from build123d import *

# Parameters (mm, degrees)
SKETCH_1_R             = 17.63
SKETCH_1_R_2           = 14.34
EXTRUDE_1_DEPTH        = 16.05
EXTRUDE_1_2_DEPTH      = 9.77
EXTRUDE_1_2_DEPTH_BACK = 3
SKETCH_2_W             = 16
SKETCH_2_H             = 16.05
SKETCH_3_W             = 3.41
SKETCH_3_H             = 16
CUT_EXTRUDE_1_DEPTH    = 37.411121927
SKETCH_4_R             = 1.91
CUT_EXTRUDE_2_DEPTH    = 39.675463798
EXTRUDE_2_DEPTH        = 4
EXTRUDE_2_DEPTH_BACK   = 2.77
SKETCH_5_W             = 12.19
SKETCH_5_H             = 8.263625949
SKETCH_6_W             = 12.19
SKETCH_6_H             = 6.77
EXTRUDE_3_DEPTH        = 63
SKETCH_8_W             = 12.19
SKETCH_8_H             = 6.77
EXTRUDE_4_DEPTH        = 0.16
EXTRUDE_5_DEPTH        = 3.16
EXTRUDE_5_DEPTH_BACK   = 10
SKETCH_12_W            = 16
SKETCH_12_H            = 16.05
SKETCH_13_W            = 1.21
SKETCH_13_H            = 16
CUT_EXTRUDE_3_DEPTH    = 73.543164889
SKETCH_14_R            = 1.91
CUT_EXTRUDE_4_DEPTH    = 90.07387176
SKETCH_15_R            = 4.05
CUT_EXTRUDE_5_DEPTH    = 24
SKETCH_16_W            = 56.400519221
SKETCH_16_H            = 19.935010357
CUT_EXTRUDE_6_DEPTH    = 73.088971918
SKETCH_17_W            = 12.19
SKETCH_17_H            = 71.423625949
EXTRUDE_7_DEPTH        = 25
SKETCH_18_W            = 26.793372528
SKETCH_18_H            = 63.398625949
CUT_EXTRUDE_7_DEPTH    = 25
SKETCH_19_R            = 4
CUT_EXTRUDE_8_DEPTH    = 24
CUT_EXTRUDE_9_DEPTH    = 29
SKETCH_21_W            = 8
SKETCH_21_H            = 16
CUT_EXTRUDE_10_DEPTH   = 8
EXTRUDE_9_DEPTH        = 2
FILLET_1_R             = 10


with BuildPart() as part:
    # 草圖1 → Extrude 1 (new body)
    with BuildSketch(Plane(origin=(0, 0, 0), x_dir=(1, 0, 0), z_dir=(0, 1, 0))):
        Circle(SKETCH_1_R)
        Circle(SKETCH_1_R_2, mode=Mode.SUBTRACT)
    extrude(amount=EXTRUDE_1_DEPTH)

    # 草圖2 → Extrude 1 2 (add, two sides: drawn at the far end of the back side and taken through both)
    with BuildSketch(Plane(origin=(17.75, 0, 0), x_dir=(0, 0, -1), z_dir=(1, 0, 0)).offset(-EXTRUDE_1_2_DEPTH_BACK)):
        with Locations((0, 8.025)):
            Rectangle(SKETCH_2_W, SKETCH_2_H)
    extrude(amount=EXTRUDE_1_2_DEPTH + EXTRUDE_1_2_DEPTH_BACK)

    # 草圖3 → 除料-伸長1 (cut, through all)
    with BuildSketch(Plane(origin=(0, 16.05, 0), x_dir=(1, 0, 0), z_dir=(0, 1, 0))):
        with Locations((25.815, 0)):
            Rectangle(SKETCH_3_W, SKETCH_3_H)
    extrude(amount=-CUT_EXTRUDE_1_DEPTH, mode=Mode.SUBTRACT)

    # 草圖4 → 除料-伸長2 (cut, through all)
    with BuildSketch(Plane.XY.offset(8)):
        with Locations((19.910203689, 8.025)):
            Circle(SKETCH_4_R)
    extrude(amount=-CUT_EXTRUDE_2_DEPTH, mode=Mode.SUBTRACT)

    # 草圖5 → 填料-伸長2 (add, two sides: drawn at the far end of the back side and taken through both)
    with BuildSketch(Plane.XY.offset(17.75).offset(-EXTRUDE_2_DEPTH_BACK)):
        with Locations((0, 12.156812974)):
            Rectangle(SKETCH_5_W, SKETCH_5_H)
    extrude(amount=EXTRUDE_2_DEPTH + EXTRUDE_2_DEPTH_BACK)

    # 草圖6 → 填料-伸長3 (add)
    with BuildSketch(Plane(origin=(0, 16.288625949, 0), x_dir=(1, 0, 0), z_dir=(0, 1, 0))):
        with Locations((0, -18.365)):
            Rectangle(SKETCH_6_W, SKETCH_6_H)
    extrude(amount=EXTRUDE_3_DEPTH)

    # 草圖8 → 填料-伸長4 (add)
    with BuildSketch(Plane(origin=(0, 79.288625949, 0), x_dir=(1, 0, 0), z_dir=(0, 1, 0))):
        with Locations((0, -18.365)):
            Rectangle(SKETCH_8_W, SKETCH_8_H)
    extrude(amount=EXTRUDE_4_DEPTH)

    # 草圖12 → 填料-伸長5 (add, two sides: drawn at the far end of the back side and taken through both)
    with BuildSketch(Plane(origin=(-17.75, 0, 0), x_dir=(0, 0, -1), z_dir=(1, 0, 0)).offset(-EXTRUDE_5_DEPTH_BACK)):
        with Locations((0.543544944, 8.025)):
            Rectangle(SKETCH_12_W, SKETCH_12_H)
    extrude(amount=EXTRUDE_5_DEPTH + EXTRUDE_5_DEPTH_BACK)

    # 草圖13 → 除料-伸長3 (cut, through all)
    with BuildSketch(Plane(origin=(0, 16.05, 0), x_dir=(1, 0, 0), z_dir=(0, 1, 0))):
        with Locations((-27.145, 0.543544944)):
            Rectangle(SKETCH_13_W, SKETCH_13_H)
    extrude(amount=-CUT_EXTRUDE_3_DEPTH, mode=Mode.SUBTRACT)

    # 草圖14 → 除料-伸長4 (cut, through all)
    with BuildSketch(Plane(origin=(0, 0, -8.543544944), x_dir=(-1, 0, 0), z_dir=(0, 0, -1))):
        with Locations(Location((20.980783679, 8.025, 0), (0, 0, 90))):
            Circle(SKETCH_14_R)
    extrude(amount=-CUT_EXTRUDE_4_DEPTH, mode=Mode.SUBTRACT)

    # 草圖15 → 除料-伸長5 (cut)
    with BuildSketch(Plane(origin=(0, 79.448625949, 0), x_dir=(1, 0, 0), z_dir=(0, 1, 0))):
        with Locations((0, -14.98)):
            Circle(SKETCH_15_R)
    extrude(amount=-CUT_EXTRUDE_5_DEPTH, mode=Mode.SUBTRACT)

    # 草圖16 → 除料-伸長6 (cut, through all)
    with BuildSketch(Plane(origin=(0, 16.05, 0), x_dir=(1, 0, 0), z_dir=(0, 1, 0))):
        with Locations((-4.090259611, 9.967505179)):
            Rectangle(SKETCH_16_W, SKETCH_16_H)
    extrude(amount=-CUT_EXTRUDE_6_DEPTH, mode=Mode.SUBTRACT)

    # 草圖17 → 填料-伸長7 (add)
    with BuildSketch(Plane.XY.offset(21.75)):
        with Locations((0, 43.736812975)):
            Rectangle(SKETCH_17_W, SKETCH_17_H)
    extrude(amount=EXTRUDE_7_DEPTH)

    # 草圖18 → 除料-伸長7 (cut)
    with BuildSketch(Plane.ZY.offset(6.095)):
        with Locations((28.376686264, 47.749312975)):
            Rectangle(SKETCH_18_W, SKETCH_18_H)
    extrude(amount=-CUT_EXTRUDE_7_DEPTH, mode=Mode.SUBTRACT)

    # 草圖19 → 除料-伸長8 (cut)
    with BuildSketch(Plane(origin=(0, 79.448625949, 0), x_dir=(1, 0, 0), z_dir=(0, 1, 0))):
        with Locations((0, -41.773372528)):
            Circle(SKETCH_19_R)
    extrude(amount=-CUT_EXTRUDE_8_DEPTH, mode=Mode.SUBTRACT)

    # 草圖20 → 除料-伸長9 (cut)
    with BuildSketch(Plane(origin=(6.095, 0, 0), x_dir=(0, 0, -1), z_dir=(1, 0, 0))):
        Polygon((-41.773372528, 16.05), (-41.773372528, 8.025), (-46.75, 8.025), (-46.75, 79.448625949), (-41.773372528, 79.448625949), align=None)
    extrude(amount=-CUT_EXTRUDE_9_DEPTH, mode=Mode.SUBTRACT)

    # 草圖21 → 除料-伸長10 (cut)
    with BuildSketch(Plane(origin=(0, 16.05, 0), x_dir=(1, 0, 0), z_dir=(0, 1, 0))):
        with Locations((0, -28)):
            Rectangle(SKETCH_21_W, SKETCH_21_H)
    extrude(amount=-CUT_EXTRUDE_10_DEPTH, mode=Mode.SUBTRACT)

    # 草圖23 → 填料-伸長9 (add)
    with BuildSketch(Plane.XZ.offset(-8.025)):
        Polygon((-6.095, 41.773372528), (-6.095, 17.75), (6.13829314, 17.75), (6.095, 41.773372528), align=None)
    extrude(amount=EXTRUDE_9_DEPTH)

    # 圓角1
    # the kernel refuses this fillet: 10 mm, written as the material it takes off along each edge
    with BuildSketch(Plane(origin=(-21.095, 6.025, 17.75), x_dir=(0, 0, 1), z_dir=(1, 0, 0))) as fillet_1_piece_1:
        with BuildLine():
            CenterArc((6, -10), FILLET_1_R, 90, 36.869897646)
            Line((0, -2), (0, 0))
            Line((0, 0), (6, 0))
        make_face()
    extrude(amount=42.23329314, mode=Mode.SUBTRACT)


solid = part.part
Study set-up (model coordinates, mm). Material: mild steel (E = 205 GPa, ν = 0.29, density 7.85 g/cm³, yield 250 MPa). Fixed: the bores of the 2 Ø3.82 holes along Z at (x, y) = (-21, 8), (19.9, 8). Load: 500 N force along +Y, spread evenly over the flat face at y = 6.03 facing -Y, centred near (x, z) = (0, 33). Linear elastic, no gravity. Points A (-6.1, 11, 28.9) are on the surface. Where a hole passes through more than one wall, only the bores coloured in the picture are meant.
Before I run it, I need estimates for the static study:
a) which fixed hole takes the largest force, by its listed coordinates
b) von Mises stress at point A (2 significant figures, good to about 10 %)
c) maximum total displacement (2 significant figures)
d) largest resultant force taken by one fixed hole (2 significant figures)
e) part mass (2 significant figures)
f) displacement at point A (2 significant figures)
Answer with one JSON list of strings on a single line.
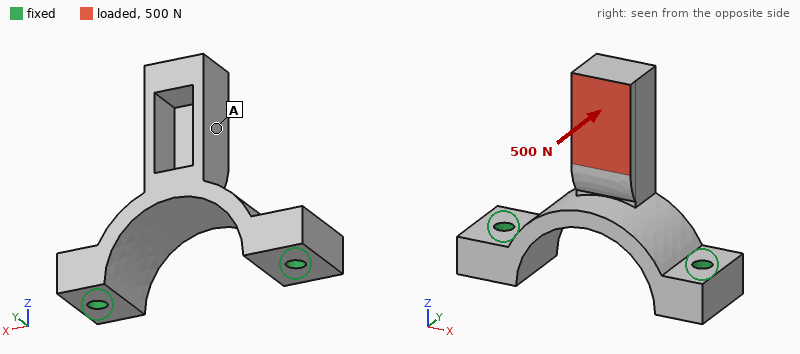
["(19.9, 8)", "22 MPa", "80 µm", "280 N", "50 g", "43 µm"]
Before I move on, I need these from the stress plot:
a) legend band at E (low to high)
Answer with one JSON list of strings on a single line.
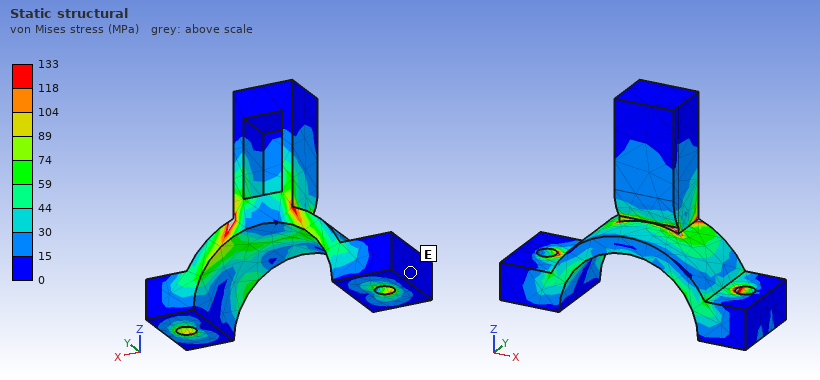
["0 to 15 MPa"]
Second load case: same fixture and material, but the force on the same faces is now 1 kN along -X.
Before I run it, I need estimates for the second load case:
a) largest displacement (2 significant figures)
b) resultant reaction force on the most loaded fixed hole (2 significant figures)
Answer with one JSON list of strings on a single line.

["63 µm", "1.1 kN"]
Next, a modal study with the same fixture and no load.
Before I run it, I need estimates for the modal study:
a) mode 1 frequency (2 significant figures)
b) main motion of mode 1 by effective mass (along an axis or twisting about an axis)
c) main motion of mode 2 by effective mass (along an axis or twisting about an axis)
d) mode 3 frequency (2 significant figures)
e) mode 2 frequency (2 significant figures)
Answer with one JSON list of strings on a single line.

["3900 Hz", "along Y", "along X", "14 kHz", "5700 Hz"]
